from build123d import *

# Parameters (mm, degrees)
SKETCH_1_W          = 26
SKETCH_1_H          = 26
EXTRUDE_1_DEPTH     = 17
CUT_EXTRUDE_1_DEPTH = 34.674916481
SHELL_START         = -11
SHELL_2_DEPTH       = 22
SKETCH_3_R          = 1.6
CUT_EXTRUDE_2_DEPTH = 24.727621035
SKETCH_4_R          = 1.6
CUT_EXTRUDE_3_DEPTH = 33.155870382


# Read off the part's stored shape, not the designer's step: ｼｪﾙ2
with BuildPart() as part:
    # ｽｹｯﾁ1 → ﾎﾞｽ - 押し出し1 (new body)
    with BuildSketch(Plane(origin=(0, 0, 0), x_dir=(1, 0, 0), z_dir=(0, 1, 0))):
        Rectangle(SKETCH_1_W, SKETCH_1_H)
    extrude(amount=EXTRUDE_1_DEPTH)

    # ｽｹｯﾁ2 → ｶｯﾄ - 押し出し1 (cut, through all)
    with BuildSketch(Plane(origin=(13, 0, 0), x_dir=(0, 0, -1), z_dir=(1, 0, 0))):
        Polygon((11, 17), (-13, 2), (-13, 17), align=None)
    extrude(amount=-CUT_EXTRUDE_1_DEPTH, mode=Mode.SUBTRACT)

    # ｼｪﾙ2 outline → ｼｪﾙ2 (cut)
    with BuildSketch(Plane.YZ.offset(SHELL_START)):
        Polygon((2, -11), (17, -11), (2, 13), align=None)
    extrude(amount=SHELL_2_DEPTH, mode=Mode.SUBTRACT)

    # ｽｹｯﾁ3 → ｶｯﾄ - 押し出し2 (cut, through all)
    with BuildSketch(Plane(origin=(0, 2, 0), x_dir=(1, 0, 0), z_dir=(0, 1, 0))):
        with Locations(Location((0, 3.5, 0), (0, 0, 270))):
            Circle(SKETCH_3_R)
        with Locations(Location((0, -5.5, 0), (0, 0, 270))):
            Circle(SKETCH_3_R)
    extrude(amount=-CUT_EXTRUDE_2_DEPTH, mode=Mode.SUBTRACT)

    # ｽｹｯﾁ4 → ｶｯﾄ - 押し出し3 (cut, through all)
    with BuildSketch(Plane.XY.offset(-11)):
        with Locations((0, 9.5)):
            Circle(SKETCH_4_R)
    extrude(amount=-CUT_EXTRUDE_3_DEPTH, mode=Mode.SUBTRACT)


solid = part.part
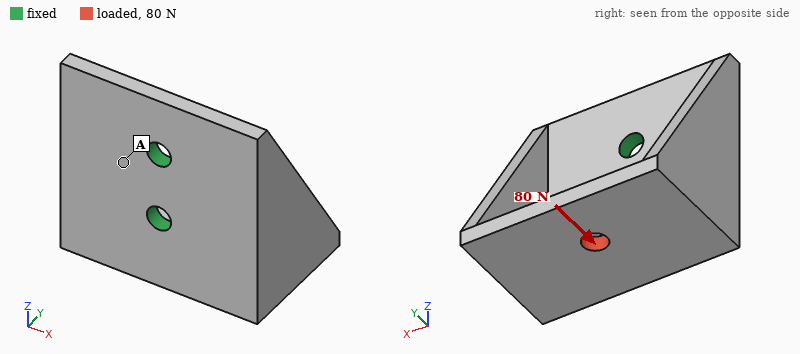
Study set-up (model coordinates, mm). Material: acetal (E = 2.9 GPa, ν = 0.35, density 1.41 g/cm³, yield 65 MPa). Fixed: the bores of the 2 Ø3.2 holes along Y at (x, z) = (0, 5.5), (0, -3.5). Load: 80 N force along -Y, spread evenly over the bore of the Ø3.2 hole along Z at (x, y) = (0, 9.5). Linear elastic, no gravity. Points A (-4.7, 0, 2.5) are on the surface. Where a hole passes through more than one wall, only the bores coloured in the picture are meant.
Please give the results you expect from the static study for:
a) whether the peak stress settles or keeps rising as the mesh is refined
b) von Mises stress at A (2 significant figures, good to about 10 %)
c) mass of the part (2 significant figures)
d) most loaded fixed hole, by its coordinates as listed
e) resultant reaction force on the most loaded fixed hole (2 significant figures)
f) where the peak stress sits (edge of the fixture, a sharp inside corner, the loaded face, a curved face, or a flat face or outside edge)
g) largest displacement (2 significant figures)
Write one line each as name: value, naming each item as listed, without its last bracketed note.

whether the peak stress settles or keeps rising as the mesh is refined: keeps rising
von Mises stress at A: 6.0 MPa
mass of the part: 4.0 g
most loaded fixed hole, by its coordinates as listed: (0, -3.5)
resultant reaction force on the most loaded fixed hole: 110 N
where the peak stress sits: edge of the fixture
largest displacement: 0.43 mm
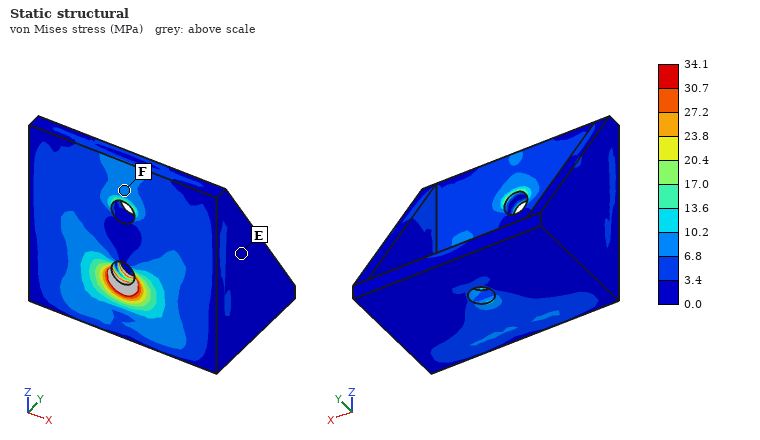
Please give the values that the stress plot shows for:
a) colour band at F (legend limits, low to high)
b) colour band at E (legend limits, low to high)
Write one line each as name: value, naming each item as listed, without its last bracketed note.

colour band at F: 6.8 to 10.2 MPa
colour band at E: 0.0 to 3.4 MPa
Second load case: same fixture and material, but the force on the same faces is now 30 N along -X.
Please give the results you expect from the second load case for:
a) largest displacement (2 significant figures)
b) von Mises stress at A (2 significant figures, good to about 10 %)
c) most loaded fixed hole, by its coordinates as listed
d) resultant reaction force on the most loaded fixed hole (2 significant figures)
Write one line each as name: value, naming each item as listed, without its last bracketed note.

largest displacement: 0.38 mm
von Mises stress at A: 5.3 MPa
most loaded fixed hole, by its coordinates as listed: (0, -3.5)
resultant reaction force on the most loaded fixed hole: 49 N
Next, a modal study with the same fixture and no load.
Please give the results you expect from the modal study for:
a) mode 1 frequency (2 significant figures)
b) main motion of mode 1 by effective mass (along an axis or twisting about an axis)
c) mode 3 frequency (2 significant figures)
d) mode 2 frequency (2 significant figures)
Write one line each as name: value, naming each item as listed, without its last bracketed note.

mode 1 frequency: 1000 Hz
main motion of mode 1 by effective mass: along X
mode 3 frequency: 2500 Hz
mode 2 frequency: 1600 Hz
